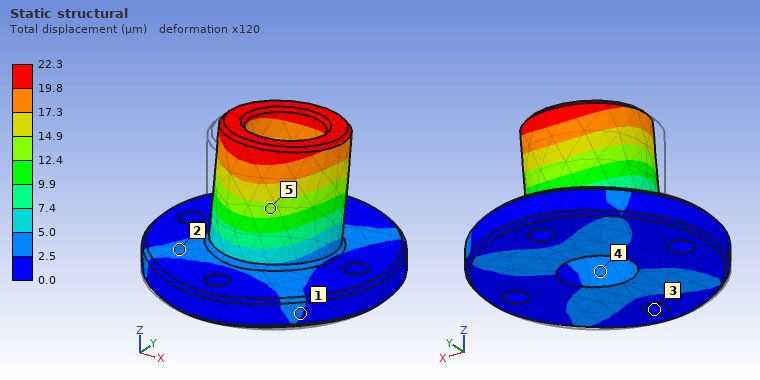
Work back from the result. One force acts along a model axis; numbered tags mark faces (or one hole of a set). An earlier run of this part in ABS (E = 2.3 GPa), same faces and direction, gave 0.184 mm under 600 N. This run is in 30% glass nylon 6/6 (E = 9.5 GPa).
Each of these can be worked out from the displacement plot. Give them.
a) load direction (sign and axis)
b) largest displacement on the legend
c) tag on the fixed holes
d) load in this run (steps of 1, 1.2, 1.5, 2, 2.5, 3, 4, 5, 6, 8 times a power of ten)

+Y
22.3 µm
3
300 N
